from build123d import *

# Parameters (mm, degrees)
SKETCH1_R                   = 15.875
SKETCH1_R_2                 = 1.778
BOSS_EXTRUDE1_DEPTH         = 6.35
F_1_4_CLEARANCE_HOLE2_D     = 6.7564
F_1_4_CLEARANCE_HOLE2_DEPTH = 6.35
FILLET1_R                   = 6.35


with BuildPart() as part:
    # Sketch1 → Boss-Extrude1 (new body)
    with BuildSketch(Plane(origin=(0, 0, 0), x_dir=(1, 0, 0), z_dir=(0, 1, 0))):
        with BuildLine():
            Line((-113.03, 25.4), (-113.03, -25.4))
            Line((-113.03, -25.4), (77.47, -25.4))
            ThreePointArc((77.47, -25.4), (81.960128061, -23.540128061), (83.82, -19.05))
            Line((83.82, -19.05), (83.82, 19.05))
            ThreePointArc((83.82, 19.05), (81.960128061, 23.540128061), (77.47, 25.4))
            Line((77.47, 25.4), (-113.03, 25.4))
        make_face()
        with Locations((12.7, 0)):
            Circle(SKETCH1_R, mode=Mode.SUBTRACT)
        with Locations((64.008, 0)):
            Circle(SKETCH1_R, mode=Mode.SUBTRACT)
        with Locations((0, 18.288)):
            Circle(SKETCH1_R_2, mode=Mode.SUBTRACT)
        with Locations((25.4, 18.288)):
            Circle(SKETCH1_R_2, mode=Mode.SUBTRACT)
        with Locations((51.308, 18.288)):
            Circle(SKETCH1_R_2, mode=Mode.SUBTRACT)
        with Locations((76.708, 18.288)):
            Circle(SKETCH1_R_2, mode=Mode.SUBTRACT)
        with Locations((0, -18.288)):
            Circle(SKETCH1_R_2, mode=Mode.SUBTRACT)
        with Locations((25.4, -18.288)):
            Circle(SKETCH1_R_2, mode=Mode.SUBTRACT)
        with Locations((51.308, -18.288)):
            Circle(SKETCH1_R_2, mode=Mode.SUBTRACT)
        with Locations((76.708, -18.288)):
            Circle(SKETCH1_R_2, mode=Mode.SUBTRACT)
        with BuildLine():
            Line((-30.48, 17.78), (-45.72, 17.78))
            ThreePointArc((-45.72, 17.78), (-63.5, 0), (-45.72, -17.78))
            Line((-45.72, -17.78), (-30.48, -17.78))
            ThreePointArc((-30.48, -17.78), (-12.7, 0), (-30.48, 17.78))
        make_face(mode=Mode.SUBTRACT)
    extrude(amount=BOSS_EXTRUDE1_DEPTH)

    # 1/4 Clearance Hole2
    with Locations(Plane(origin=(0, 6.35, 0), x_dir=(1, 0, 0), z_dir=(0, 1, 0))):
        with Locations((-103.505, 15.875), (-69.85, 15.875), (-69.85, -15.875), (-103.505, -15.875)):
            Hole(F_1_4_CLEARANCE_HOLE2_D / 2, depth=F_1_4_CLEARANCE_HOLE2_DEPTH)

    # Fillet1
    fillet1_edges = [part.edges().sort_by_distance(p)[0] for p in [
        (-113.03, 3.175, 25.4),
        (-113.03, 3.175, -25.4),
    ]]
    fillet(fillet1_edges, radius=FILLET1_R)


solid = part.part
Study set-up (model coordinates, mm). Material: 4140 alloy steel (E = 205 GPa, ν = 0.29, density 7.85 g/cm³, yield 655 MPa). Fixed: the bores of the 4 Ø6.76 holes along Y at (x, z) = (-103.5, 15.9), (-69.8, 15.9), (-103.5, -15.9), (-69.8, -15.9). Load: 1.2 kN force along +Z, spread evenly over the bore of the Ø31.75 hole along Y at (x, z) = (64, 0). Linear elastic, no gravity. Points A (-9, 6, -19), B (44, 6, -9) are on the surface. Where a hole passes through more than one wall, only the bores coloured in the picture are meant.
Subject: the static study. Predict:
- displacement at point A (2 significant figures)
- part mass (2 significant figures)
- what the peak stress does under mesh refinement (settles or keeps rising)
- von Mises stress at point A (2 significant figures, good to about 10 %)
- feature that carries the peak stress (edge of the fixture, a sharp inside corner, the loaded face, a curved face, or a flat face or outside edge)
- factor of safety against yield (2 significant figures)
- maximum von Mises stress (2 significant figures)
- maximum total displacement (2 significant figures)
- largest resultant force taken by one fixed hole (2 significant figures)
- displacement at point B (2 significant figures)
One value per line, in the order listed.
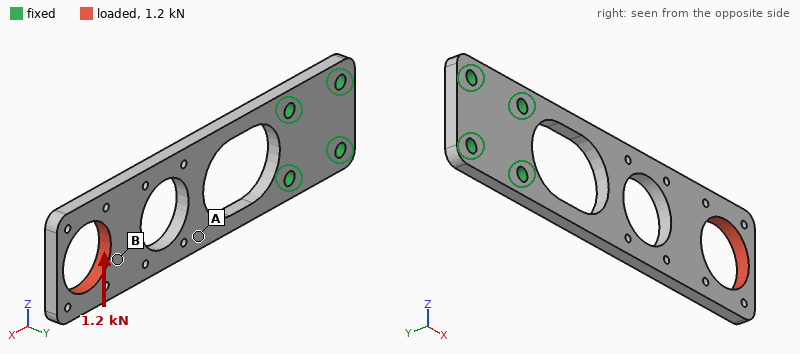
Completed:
0.10 mm
330 g
settles
33 MPa
a flat face or outside edge
3.9
170 MPa
0.23 mm
3.4 kN
0.17 mm
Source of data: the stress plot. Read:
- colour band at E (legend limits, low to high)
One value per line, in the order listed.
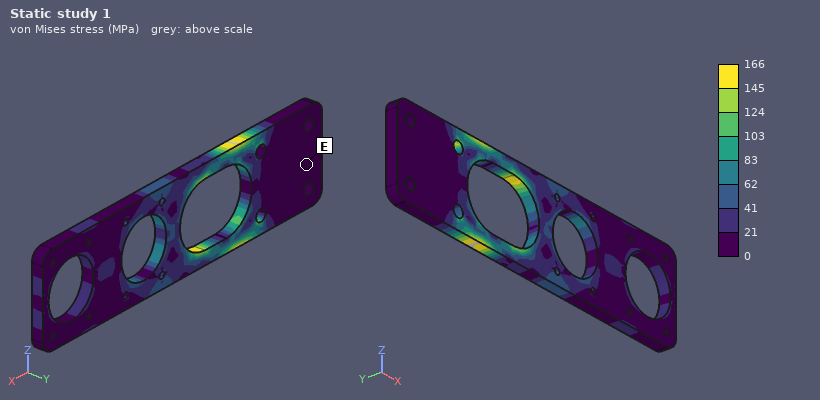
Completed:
0 to 21 MPa
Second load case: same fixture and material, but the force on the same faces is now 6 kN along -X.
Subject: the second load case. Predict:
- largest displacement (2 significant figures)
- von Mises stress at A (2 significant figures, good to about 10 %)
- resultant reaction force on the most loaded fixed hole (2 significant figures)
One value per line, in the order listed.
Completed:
47 µm
34 MPa
2.8 kN
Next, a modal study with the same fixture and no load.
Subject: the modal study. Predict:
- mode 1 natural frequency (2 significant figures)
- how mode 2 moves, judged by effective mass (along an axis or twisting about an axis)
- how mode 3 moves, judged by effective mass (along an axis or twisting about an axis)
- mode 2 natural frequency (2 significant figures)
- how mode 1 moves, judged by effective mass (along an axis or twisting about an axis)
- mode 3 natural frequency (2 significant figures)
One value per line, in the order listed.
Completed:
180 Hz
twisting about X
along Z
940 Hz
along Y
1100 Hz
